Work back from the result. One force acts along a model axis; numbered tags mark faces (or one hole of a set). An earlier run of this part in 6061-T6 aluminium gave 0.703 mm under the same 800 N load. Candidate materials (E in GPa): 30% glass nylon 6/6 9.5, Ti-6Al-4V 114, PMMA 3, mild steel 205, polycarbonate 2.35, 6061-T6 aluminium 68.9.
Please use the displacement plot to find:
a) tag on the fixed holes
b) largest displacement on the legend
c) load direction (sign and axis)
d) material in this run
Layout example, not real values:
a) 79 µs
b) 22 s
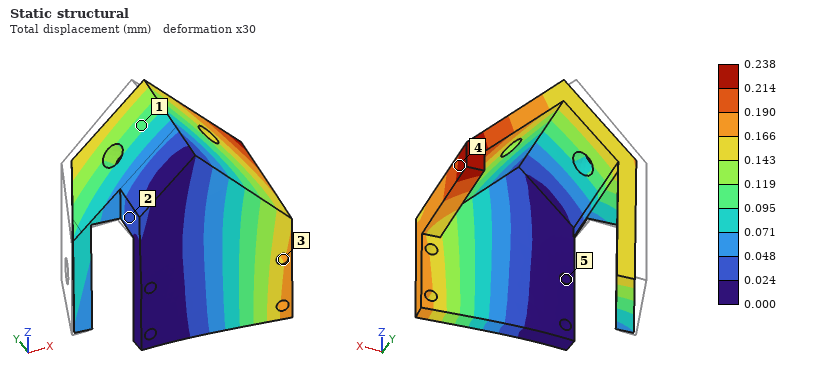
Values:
a) 5
b) 0.238 mm
c) -Y
d) mild steel
